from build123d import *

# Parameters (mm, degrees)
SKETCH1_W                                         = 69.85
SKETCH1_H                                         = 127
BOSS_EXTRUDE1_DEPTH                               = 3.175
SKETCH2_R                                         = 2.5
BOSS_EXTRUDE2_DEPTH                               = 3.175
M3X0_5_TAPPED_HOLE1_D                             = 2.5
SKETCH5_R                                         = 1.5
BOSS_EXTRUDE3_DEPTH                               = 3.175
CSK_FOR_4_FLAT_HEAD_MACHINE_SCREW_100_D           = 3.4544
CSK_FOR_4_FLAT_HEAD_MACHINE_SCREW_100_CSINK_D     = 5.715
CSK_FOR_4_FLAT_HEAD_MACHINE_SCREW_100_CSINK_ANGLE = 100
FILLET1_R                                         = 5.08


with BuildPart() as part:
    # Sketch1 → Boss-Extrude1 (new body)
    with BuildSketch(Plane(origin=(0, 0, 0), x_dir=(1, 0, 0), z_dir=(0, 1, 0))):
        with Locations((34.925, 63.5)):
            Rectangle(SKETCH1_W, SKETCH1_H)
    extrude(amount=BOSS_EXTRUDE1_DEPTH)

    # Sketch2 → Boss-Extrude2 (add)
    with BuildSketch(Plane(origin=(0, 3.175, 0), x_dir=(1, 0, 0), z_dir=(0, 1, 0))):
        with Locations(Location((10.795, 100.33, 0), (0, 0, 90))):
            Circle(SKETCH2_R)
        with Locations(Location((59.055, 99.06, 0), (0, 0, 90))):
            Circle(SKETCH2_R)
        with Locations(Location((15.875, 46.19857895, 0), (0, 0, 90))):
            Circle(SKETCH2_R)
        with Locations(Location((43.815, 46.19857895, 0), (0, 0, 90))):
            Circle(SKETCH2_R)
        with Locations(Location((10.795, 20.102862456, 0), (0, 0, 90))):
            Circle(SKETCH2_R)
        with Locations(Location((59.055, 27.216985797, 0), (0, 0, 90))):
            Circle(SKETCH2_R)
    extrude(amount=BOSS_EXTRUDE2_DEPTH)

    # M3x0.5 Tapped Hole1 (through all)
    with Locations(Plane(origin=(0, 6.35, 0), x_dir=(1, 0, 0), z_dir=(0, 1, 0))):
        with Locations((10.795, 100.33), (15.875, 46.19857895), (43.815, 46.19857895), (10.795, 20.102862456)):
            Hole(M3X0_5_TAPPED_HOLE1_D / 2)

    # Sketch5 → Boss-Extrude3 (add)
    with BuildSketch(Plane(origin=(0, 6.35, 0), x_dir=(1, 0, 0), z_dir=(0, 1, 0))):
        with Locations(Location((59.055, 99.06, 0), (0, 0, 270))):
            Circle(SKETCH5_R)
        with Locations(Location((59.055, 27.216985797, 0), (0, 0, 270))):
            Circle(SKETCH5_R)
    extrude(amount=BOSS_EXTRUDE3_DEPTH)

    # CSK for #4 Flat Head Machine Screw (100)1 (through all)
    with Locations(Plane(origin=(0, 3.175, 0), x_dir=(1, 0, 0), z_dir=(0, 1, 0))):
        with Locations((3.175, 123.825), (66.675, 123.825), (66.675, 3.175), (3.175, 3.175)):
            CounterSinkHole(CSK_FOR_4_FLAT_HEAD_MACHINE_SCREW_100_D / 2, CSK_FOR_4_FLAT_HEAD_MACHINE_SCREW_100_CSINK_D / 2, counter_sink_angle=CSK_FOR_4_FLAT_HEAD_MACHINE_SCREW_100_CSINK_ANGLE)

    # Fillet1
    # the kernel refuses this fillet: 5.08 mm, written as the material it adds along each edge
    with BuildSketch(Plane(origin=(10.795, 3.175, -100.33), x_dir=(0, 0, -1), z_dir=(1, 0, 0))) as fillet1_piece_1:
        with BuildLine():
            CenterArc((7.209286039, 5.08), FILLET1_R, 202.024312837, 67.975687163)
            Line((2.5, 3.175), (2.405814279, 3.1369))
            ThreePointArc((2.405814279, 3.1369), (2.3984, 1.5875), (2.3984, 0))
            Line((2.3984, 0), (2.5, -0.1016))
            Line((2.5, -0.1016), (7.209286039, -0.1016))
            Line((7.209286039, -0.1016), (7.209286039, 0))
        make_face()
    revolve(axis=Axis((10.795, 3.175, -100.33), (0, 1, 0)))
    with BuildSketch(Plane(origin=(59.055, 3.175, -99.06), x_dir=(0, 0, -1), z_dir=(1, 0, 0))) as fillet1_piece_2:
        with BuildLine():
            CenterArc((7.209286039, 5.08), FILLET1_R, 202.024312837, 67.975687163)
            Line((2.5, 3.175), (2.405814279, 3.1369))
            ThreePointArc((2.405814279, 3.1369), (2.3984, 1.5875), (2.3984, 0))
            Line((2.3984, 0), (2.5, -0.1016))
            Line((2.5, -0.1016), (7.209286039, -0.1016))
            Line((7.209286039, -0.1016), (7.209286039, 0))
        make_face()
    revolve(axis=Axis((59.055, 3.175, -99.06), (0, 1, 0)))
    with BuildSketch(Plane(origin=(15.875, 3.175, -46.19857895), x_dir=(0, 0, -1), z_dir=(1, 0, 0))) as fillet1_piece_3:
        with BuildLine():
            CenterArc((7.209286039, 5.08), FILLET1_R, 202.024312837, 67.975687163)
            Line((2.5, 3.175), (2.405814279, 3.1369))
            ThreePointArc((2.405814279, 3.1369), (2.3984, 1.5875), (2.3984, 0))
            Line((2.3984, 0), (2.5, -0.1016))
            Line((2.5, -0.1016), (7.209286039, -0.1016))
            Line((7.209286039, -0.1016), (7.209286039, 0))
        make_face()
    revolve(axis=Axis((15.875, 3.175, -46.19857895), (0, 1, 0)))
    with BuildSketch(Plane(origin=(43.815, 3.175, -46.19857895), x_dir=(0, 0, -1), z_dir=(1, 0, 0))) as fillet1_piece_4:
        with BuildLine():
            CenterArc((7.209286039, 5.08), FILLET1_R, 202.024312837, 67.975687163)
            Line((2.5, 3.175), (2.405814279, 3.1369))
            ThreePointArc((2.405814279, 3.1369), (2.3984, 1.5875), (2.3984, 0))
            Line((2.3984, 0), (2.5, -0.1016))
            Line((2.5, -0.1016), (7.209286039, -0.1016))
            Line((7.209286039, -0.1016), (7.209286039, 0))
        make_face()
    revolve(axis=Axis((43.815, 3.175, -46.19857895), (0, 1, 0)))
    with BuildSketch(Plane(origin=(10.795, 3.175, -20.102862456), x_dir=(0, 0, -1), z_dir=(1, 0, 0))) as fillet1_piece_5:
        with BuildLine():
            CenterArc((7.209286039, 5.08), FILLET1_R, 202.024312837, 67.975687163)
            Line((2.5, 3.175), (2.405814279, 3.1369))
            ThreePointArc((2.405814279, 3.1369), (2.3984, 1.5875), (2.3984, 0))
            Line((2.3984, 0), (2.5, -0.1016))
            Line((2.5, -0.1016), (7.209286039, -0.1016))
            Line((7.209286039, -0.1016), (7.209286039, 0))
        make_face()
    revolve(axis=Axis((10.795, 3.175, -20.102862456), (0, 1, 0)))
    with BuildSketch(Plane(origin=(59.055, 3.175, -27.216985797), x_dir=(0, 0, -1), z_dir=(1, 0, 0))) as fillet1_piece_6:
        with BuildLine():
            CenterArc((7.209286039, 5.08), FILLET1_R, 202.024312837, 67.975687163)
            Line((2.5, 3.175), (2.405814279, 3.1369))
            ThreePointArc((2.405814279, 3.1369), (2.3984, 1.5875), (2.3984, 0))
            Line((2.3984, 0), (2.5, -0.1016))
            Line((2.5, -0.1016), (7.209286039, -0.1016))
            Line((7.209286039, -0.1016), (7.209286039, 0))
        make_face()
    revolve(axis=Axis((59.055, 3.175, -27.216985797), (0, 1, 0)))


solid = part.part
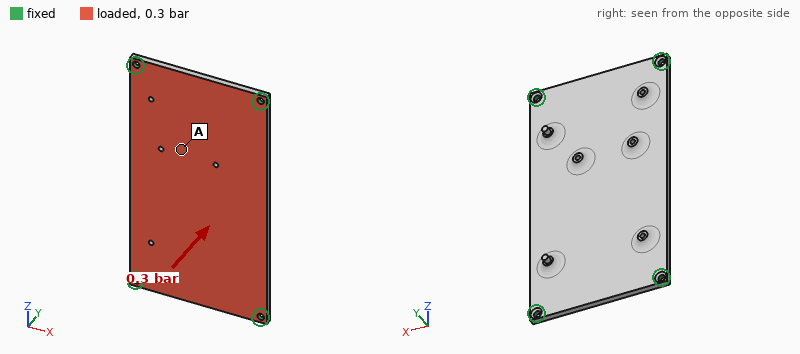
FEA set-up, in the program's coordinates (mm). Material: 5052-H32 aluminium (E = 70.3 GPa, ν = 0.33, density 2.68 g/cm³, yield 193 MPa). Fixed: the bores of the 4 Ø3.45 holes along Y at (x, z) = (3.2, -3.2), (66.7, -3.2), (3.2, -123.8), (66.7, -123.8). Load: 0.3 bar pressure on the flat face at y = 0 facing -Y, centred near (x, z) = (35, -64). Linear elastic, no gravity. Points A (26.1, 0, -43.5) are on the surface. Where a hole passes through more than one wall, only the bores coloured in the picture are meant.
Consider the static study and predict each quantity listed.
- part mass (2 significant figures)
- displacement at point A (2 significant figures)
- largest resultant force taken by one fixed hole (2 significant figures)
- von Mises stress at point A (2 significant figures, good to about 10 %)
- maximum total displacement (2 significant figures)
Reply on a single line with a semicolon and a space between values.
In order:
77 g; 0.12 mm; 81 N; 8.1 MPa; 0.15 mm
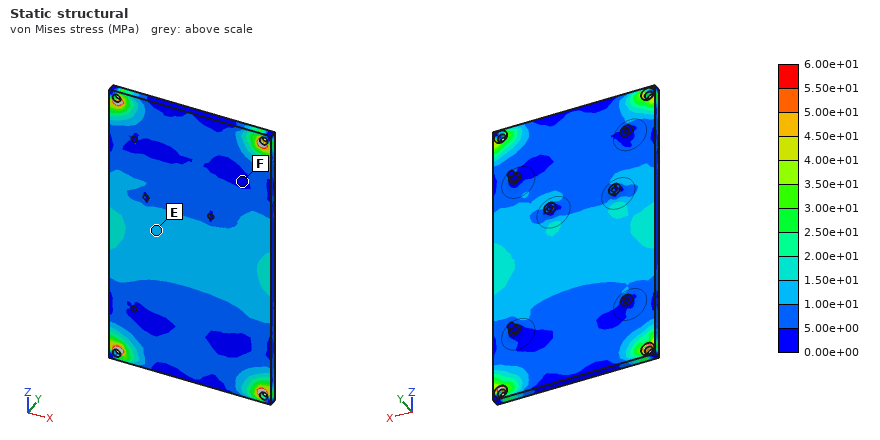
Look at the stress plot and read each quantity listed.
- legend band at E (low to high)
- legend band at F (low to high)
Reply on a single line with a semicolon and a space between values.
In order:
1.00e+01 to 1.50e+01 MPa; 0.00e+00 to 5.00e+00 MPa
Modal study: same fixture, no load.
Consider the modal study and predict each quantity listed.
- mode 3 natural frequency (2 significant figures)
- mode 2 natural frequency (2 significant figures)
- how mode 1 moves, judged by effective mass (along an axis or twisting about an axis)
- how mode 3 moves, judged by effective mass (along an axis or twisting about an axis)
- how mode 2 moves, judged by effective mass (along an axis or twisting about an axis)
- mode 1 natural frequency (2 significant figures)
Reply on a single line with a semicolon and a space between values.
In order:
2500 Hz; 1700 Hz; along Y; twisting about X; twisting about Z; 870 Hz
